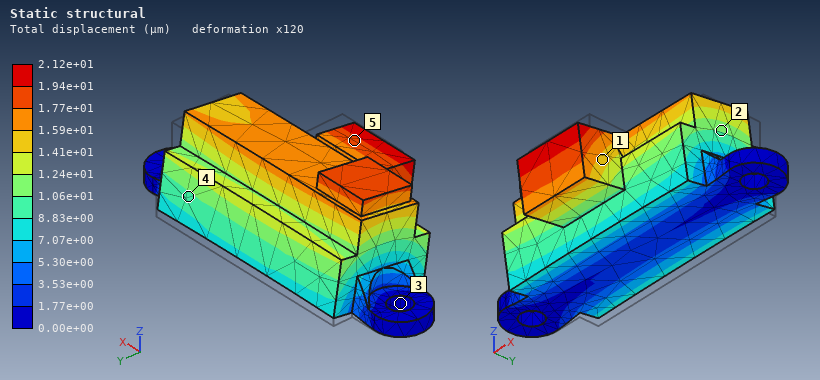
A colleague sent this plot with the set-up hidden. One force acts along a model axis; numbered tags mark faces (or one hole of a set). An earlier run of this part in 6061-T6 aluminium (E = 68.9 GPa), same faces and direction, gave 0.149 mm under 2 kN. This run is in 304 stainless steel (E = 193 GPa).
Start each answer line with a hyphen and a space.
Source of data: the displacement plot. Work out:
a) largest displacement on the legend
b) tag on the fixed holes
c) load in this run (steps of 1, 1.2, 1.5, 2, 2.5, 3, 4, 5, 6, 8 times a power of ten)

- 2.12e+01 µm
- 3
- 800 N
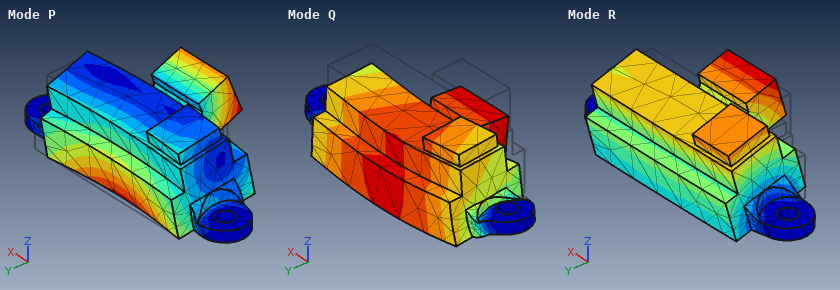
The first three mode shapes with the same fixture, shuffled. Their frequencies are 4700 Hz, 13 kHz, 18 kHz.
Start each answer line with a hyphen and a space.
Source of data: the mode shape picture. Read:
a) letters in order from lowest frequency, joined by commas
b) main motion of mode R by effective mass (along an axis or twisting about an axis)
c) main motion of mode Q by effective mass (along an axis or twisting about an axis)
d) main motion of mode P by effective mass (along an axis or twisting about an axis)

- R, Q, P
- along Y
- along Z
- along Y
